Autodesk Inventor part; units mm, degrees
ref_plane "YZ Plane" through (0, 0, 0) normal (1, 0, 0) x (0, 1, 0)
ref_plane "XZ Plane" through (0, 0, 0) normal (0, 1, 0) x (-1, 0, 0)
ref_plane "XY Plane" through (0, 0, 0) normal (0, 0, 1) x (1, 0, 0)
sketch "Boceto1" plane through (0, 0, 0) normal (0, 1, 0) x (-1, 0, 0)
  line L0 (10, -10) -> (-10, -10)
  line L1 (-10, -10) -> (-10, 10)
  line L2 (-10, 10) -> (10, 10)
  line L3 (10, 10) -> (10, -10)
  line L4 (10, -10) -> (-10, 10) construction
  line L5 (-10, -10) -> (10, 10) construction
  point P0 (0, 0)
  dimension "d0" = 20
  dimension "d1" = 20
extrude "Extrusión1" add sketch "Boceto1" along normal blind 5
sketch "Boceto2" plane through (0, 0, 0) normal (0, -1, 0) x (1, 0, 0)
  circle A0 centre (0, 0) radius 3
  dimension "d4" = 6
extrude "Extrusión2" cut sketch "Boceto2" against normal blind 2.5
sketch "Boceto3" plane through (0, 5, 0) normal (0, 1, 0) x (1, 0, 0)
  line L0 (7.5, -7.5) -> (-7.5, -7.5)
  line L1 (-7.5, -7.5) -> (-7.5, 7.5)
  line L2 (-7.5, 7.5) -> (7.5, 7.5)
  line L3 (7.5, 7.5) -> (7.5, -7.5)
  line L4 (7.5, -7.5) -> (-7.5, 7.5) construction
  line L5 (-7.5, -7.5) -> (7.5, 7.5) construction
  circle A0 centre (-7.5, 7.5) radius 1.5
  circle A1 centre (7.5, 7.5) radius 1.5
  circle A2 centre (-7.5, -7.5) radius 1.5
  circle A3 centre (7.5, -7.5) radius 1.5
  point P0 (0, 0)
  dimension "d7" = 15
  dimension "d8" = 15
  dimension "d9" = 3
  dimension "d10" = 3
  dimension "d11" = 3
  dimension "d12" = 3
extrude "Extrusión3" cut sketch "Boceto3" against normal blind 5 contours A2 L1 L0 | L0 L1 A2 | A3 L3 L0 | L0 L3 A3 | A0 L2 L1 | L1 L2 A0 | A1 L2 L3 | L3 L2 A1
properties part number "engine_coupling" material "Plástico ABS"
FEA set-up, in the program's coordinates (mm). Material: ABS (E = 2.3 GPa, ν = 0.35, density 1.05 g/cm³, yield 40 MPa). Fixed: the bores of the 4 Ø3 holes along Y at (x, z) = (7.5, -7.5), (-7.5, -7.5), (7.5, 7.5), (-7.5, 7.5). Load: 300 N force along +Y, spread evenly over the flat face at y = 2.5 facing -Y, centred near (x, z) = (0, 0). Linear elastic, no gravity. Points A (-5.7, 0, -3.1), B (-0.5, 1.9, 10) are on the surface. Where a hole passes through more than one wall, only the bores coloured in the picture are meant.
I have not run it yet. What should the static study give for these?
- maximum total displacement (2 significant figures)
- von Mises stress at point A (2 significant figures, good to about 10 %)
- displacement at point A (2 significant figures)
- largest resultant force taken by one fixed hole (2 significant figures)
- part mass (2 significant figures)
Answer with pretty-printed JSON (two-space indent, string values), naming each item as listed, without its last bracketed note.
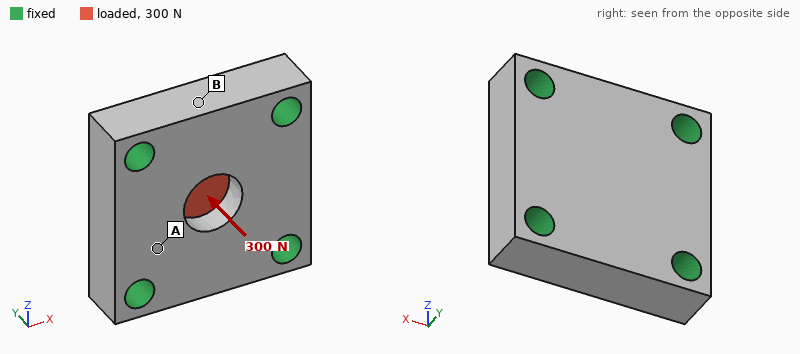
{
  "maximum total displacement": "77 µm",
  "von Mises stress at point A": "5.2 MPa",
  "displacement at point A": "22 µm",
  "largest resultant force taken by one fixed hole": "77 N",
  "part mass": "1.9 g"
}
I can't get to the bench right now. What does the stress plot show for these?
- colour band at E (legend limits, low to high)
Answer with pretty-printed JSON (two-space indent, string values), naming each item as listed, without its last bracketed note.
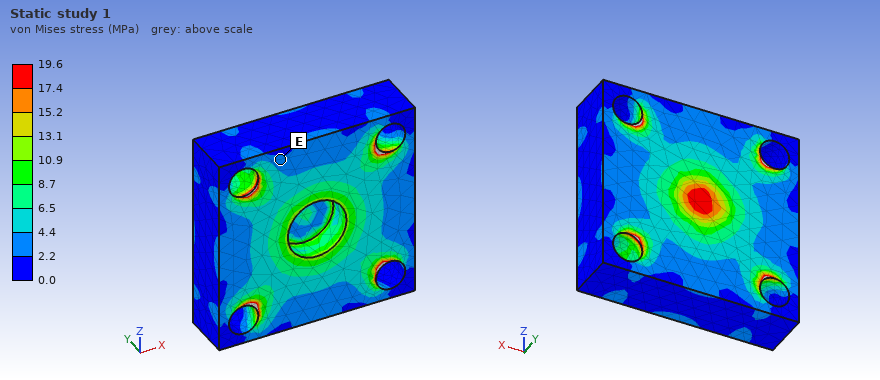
{
  "colour band at E": "2.2 to 4.4 MPa"
}
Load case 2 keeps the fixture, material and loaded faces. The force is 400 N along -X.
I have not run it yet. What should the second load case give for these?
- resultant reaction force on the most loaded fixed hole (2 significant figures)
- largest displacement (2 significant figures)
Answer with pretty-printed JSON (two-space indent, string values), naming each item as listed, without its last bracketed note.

{
  "resultant reaction force on the most loaded fixed hole": "110 N",
  "largest displacement": "46 µm"
}
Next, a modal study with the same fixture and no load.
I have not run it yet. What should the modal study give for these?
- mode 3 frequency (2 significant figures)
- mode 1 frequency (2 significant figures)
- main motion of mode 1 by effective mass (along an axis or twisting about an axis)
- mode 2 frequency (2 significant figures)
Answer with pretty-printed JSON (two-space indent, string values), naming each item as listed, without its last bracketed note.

{
  "mode 3 frequency": "27 kHz",
  "mode 1 frequency": "19 kHz",
  "main motion of mode 1 by effective mass": "along Y",
  "mode 2 frequency": "27 kHz"
}
